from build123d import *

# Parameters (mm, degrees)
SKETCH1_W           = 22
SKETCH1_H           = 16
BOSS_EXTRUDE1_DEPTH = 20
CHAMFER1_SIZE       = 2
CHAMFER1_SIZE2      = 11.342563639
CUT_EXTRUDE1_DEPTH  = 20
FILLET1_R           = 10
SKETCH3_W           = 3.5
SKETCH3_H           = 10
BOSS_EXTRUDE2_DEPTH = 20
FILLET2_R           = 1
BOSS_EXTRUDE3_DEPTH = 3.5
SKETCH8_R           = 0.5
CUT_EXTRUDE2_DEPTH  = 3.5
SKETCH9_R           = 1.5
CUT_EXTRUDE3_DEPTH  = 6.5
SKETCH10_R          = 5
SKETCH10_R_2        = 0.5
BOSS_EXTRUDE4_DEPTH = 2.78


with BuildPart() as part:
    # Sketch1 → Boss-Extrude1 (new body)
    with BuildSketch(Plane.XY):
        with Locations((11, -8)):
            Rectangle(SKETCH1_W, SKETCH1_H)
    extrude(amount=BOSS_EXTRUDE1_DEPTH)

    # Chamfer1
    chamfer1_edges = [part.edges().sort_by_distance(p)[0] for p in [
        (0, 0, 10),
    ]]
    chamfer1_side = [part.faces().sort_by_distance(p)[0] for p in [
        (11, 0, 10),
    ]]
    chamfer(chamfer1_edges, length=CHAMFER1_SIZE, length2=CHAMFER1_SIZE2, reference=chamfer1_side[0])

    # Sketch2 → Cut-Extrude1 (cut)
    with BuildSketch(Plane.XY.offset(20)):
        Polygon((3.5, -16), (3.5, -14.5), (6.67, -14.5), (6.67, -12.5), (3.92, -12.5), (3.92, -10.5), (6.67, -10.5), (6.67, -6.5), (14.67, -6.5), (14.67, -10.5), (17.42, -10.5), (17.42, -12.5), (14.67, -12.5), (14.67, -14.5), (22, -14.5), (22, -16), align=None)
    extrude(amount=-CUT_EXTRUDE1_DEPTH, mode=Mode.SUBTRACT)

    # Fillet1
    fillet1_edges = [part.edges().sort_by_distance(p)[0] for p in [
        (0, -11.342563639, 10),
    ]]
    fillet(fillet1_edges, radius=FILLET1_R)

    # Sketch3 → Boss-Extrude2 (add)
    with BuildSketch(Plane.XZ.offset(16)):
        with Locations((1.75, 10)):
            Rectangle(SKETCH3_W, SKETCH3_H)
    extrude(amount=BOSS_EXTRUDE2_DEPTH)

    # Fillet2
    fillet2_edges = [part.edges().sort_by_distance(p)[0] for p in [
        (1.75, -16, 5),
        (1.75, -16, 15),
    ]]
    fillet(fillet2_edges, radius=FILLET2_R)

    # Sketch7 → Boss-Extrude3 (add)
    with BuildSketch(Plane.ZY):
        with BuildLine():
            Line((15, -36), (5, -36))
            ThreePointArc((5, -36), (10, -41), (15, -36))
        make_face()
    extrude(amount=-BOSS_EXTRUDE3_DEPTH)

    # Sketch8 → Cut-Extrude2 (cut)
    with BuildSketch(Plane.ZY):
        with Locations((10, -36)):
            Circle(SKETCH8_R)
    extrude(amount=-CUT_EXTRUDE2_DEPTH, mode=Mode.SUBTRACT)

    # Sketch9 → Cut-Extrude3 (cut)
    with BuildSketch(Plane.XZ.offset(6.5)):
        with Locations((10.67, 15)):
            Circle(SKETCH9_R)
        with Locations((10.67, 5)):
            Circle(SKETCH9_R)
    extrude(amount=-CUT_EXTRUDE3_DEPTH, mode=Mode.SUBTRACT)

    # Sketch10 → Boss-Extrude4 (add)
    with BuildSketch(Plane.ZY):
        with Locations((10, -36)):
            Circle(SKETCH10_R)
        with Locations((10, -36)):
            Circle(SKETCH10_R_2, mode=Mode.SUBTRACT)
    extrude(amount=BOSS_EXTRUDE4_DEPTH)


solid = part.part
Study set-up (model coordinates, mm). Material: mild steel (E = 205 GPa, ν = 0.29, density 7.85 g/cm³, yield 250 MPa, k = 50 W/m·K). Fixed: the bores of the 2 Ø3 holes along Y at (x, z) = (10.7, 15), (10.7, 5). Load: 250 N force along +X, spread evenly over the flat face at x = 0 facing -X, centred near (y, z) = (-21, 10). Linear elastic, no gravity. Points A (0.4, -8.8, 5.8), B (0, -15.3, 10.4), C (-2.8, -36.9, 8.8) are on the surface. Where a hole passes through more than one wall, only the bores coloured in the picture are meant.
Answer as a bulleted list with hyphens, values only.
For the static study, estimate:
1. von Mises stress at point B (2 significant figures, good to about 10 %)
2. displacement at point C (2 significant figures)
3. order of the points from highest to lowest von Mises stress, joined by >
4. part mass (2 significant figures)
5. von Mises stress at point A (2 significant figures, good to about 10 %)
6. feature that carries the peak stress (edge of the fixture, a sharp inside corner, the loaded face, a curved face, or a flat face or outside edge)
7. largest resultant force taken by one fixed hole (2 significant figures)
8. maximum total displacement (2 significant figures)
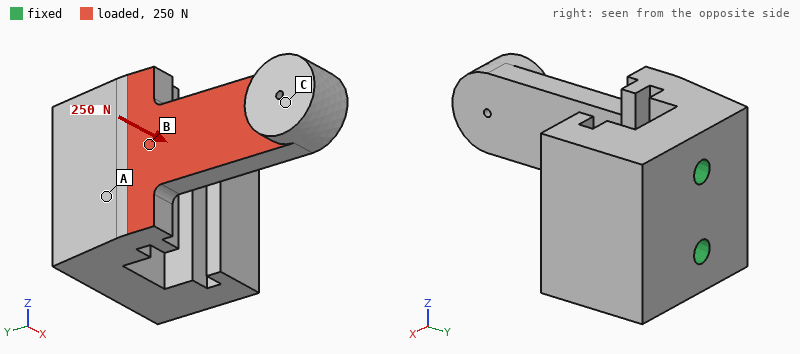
- 56 MPa
- 61 µm
- B > A > C
- 45 g
- 41 MPa
- the loaded face
- 130 N
- 71 µm
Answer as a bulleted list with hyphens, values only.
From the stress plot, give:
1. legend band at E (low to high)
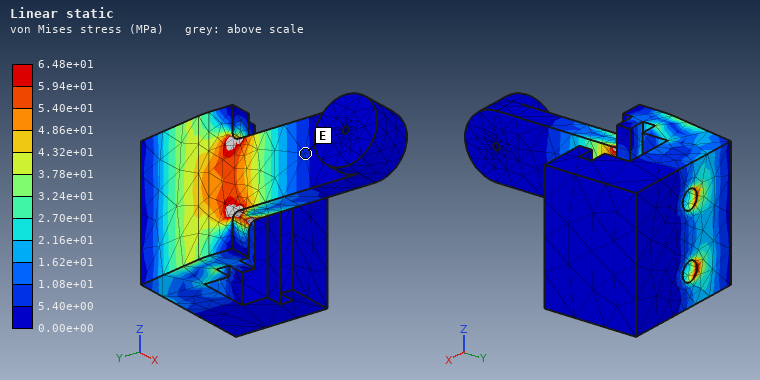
- 5.40e+00 to 1.08e+01 MPa
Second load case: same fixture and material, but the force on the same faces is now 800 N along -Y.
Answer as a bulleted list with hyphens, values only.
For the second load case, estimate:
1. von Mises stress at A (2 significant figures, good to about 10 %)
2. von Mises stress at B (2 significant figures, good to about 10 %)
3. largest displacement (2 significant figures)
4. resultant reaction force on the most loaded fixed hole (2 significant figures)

- 40 MPa
- 51 MPa
- 65 µm
- 400 N
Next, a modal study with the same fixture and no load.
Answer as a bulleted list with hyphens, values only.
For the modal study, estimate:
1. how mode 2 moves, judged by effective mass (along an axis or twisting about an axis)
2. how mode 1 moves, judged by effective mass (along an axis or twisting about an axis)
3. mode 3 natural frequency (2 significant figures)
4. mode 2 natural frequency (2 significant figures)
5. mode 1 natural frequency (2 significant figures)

- along Z
- along X
- 13 kHz
- 6700 Hz
- 2600 Hz
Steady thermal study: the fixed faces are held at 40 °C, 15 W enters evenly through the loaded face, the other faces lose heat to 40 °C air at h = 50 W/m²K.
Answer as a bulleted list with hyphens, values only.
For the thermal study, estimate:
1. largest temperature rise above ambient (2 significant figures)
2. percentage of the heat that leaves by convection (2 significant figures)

- 78 K
- 21 %
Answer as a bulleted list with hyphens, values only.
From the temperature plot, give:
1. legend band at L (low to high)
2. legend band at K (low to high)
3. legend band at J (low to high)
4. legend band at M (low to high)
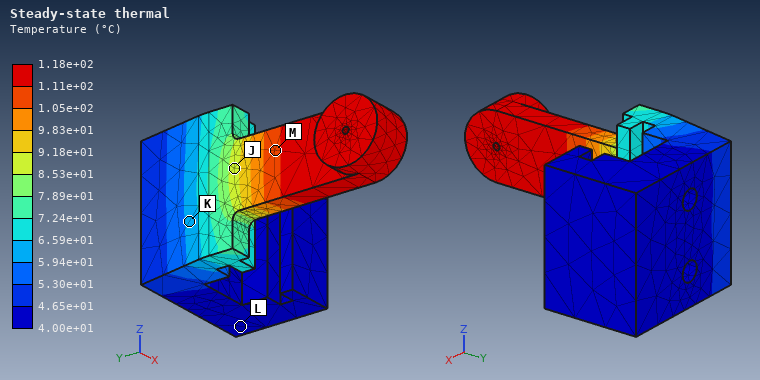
- 4.00e+01 to 4.65e+01 °C
- 5.94e+01 to 6.59e+01 °C
- 8.53e+01 to 9.18e+01 °C
- 1.05e+02 to 1.11e+02 °C
